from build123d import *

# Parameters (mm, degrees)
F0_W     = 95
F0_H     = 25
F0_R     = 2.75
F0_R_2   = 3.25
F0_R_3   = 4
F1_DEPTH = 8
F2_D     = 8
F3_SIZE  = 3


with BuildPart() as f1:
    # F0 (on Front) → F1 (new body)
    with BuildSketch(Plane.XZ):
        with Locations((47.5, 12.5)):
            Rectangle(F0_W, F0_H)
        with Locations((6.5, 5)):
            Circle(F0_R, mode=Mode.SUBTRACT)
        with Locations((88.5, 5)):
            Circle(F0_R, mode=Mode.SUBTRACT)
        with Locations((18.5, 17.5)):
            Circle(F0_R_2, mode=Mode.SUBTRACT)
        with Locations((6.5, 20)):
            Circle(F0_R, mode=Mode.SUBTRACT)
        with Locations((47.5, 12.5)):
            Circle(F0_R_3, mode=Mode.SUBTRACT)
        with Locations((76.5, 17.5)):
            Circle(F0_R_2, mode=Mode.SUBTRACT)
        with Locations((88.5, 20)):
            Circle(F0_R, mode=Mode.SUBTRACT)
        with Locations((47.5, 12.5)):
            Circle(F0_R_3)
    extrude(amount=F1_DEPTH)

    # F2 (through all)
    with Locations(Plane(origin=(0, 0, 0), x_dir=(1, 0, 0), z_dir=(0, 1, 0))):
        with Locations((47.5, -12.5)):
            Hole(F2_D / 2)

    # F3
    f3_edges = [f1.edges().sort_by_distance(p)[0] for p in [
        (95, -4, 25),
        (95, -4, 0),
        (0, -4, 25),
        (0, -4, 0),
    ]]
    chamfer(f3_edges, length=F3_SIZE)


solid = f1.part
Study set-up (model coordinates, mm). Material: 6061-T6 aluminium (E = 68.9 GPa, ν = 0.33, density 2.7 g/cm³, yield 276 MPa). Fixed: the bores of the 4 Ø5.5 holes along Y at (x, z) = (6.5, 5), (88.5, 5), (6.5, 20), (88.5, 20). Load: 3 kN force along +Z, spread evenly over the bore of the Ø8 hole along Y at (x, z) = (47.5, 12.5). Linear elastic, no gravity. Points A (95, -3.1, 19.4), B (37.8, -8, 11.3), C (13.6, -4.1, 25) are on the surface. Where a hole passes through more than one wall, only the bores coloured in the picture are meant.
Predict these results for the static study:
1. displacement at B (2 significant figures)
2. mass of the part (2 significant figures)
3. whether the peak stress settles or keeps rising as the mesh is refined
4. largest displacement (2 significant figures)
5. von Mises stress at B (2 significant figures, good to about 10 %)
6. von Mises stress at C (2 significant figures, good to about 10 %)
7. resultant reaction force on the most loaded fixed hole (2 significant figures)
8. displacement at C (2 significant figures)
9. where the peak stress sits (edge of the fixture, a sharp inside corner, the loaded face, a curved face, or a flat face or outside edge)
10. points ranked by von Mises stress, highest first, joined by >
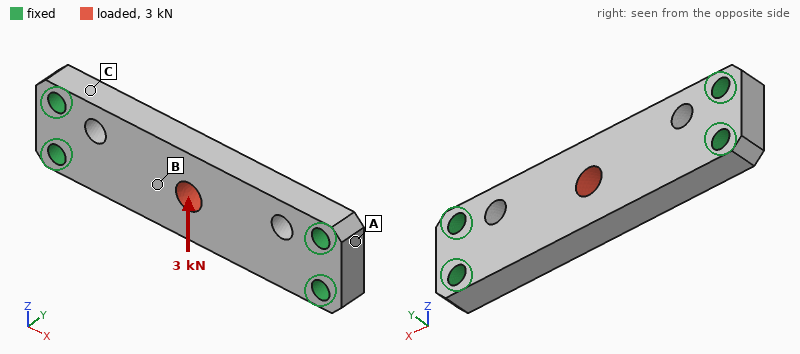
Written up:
22 µm
46 g
keeps rising
27 µm
17 MPa
33 MPa
1.8 kN
4.7 µm
edge of the fixture
C > B > A
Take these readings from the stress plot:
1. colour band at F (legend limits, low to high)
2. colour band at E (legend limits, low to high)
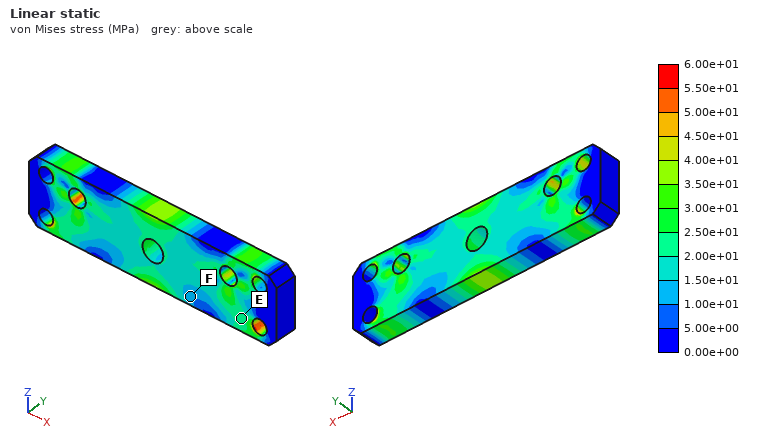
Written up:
1.00e+01 to 1.50e+01 MPa
2.00e+01 to 2.50e+01 MPa
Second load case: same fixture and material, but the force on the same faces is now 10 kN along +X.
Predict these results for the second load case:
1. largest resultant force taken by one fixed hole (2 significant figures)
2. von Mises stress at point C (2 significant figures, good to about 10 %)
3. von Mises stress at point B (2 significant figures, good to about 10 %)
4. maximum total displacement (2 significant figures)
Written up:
2.8 kN
33 MPa
41 MPa
19 µm
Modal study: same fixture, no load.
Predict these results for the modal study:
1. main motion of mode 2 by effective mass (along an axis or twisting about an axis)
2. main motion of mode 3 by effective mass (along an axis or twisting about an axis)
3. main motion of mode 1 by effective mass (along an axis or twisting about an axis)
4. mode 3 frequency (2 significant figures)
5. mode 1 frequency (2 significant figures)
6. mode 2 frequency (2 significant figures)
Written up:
twisting about X
along Z
along Y
13 kHz
6000 Hz
12 kHz
